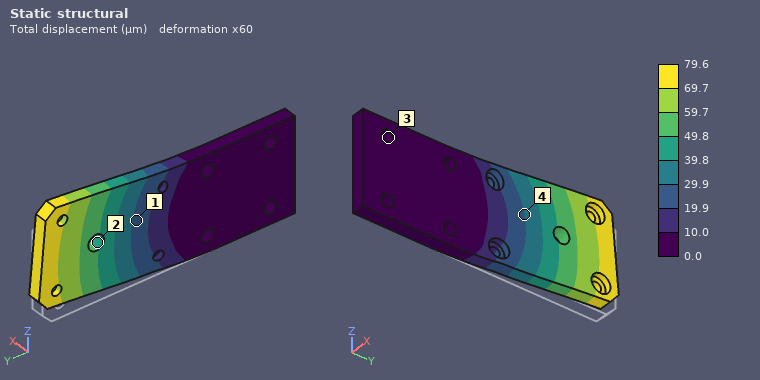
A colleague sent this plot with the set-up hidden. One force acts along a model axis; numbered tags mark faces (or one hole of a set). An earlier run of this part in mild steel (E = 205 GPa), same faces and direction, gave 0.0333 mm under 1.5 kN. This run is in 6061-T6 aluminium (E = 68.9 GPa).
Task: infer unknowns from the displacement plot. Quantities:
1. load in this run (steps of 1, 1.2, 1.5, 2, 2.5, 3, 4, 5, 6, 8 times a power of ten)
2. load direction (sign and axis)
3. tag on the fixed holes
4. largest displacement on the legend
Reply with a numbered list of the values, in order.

1. 1.2 kN
2. +Z
3. 3
4. 79.6 µm
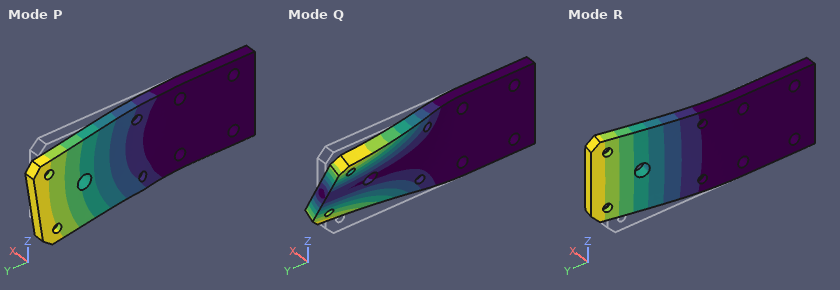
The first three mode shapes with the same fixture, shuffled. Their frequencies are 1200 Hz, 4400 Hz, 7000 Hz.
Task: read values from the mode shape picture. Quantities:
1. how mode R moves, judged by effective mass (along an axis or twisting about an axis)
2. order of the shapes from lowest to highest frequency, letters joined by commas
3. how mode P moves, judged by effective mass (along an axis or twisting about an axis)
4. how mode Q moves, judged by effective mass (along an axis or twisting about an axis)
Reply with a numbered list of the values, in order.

1. along X
2. R, Q, P
3. along Z
4. twisting about Y
